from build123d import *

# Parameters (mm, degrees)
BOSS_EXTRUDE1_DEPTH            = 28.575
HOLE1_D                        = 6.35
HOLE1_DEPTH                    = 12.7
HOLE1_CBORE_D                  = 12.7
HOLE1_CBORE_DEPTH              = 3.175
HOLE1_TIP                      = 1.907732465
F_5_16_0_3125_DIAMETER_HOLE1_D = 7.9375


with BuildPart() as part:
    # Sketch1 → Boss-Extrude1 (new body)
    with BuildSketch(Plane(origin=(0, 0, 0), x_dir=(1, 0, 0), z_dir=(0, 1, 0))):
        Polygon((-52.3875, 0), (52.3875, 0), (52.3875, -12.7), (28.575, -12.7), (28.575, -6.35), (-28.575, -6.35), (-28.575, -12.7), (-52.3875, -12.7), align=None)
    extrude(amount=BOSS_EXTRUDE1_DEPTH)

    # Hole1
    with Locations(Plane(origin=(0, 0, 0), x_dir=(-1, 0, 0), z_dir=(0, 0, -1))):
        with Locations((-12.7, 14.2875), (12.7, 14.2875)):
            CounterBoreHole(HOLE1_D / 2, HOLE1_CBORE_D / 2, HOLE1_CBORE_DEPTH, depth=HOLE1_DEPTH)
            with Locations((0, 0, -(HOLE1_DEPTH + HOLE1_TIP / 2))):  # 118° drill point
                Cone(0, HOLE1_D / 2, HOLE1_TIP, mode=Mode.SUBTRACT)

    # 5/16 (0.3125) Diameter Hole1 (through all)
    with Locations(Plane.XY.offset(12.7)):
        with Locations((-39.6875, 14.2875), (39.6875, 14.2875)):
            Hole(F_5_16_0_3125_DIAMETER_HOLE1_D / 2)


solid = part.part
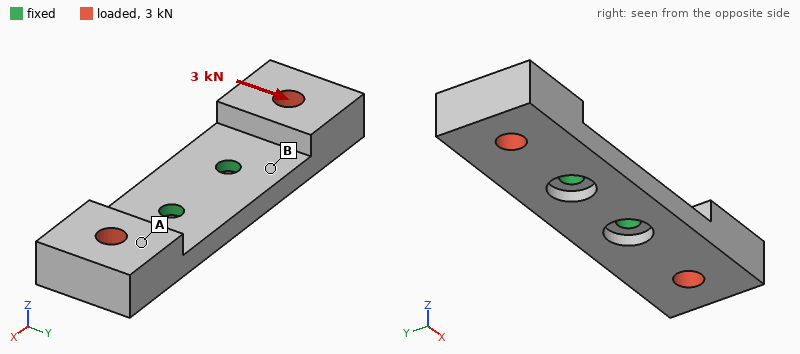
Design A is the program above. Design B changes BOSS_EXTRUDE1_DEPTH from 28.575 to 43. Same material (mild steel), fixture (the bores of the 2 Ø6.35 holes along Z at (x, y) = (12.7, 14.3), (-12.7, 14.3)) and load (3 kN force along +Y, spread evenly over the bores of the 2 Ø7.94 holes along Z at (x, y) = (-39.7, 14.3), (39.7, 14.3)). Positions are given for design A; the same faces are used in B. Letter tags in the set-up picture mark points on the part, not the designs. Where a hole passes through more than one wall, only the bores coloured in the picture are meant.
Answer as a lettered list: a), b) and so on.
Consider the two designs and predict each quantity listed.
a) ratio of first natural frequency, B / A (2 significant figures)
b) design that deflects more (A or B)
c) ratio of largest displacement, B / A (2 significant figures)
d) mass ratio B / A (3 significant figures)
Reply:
a) 0.88
b) A
c) 0.57
d) 1.55
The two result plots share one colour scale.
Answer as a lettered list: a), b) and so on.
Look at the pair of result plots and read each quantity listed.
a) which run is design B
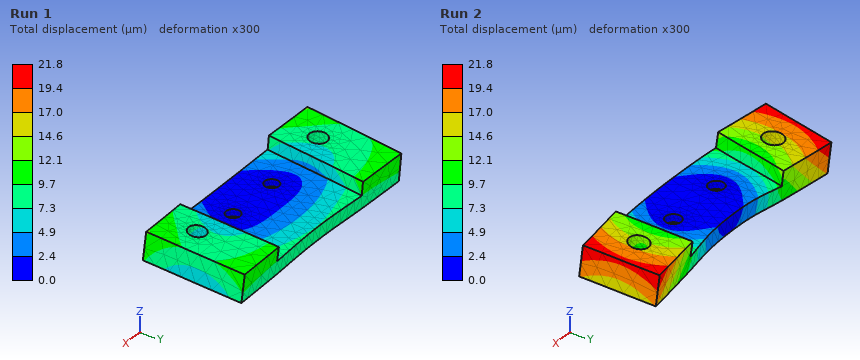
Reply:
a) Run 1
